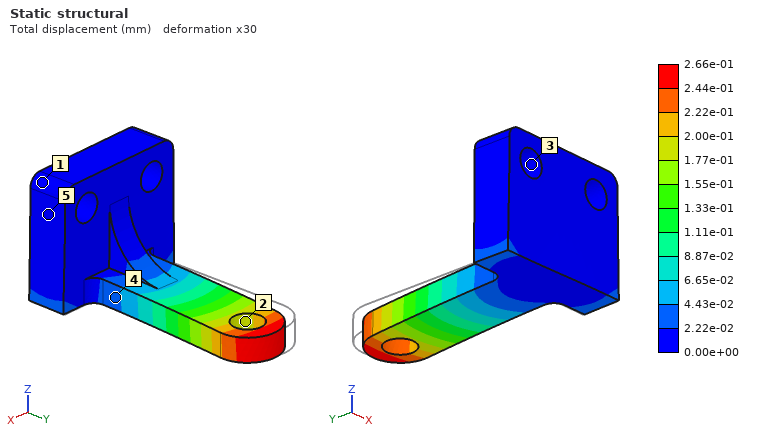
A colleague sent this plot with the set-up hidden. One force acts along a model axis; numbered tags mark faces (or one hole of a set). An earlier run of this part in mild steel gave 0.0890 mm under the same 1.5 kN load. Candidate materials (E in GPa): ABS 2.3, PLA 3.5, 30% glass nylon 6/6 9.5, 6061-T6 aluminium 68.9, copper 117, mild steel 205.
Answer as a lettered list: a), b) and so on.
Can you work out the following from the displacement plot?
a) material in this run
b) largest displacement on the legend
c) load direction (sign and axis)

a) 6061-T6 aluminium
b) 2.66e-01 mm
c) +X
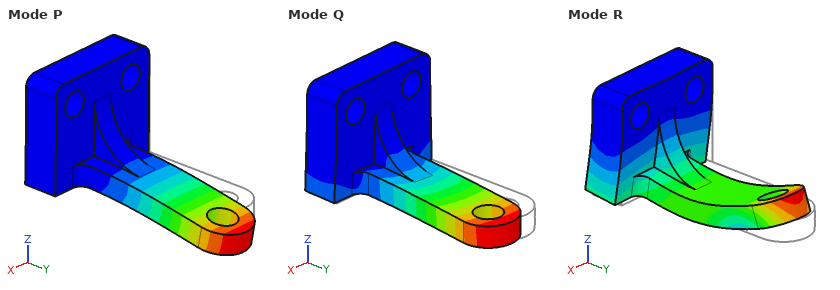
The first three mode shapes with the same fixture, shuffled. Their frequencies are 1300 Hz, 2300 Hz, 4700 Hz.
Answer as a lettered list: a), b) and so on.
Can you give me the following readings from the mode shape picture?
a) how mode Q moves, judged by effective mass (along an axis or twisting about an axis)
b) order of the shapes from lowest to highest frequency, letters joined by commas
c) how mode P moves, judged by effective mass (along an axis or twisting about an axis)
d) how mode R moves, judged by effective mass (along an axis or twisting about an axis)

a) along X
b) P, Q, R
c) along Z
d) along Y
